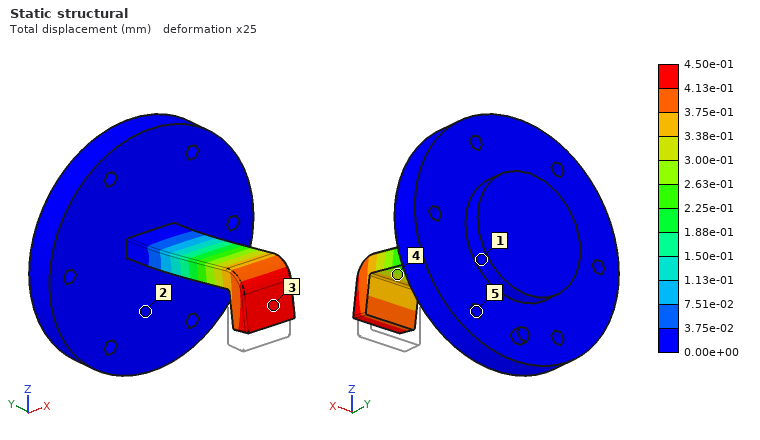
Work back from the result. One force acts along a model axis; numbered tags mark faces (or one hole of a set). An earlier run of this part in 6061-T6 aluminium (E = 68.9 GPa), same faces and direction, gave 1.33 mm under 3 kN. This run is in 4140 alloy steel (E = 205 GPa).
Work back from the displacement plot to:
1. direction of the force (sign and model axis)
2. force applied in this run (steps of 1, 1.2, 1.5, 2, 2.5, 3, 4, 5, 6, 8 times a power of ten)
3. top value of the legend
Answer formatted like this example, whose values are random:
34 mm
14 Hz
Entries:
+Z
3 kN
4.50e-01 mm
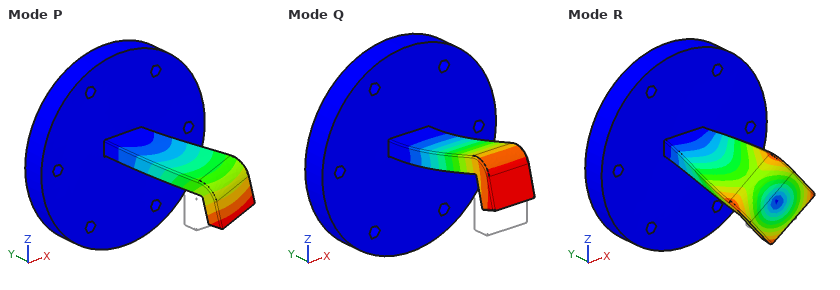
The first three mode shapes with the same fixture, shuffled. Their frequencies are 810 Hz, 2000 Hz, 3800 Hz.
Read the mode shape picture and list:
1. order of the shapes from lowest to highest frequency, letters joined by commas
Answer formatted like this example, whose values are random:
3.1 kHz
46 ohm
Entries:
Q, P, R
